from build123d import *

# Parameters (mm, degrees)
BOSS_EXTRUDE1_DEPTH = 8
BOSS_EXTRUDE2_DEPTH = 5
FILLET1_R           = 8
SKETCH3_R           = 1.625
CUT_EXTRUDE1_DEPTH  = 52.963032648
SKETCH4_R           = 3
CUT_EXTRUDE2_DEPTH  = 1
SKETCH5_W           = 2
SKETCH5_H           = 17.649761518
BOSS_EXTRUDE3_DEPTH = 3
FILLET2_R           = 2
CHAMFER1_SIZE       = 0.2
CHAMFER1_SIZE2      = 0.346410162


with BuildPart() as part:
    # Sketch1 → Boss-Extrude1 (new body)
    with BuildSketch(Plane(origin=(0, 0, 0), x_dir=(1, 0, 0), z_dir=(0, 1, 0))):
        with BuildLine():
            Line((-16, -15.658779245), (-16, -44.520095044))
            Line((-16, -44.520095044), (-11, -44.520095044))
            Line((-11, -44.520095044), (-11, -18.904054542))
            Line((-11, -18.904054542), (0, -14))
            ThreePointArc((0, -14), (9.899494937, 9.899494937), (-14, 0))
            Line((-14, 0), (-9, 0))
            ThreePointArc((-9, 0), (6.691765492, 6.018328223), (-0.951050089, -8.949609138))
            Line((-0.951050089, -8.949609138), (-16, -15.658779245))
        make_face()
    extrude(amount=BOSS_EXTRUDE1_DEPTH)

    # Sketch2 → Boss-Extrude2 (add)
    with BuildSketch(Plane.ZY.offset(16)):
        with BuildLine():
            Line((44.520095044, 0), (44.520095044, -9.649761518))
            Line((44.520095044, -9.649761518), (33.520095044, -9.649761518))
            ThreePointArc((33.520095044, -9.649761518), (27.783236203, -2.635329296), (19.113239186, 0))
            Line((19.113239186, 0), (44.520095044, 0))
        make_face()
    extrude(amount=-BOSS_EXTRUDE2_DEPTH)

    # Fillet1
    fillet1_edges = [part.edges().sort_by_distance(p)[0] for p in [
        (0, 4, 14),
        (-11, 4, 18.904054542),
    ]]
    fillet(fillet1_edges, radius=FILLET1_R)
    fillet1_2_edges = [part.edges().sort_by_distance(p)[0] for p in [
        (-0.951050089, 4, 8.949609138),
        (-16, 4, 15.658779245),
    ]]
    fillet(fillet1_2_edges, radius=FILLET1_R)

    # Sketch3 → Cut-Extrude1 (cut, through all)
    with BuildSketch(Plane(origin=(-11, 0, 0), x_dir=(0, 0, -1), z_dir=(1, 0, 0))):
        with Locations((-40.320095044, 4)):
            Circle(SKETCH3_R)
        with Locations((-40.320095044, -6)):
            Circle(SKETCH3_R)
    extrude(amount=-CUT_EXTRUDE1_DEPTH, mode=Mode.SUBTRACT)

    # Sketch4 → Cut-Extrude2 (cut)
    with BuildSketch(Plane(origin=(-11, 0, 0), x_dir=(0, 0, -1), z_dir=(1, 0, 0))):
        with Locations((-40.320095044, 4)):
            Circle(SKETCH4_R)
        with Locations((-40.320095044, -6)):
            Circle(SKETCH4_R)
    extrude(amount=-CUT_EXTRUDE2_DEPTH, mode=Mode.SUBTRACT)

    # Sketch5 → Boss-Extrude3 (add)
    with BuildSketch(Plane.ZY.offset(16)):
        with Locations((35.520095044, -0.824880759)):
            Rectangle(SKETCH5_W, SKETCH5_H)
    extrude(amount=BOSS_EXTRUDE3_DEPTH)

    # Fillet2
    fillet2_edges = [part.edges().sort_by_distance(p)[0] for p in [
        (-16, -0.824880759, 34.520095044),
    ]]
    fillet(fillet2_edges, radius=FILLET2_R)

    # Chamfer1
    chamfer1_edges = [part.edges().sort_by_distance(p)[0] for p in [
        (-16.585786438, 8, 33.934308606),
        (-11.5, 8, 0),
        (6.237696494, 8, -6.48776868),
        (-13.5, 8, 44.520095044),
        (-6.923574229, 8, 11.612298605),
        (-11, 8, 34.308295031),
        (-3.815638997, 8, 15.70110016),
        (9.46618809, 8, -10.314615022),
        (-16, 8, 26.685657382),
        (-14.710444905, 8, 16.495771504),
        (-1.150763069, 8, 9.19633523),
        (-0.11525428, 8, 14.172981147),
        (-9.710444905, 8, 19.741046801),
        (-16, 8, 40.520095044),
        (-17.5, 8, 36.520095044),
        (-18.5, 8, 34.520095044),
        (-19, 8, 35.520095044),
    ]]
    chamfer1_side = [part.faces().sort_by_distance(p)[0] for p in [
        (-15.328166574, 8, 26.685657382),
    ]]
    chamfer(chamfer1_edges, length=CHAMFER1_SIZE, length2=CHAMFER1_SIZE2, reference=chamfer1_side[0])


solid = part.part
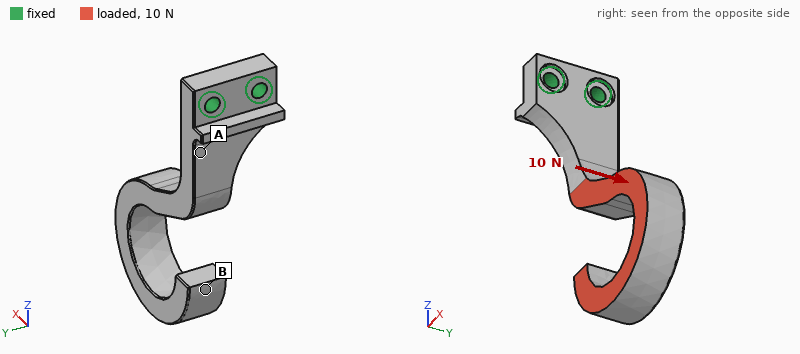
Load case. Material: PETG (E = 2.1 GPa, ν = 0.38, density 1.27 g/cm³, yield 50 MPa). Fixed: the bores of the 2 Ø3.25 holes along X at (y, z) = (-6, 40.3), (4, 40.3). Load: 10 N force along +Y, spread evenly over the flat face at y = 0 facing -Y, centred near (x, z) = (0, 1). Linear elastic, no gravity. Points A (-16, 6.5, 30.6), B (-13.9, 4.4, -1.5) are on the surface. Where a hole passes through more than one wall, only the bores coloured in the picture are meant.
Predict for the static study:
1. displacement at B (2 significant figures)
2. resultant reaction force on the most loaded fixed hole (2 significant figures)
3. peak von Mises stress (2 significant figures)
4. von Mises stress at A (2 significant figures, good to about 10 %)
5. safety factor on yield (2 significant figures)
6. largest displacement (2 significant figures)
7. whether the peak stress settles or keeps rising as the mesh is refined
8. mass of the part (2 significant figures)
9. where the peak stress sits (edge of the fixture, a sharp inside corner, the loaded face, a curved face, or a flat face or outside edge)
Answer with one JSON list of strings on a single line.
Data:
["0.55 mm", "37 N", "7.6 MPa", "3.3 MPa", "6.5", "0.81 mm", "settles", "5.8 g", "a curved face"]
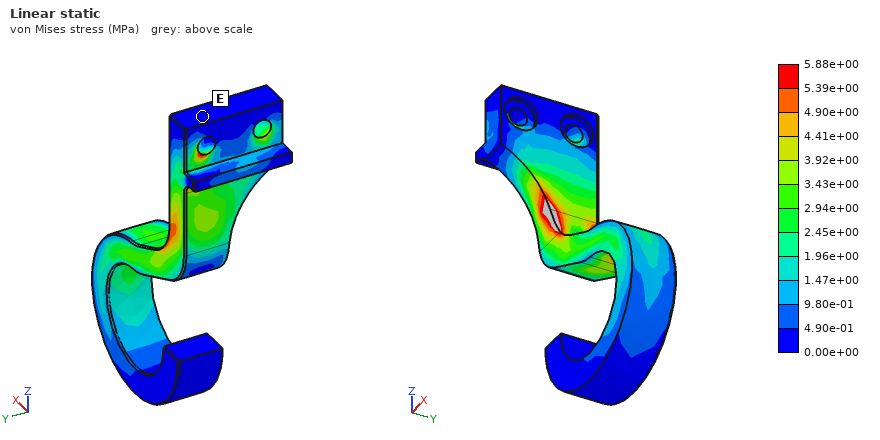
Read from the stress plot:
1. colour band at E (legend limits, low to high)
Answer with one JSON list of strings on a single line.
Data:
["0.00e+00 to 4.90e-01 MPa"]
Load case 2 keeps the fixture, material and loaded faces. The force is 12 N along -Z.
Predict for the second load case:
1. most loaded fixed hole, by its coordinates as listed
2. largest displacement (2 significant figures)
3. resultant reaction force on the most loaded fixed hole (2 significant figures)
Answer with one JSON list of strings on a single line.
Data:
["(4, 40.3)", "0.81 mm", "7.0 N"]
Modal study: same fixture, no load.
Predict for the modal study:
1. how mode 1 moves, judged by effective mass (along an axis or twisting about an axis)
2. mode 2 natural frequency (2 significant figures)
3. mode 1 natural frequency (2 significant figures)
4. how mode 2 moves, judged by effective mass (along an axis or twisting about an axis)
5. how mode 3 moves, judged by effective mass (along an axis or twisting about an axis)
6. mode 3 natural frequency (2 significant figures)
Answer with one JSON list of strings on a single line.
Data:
["along X", "340 Hz", "230 Hz", "along Y", "along Z", "620 Hz"]
